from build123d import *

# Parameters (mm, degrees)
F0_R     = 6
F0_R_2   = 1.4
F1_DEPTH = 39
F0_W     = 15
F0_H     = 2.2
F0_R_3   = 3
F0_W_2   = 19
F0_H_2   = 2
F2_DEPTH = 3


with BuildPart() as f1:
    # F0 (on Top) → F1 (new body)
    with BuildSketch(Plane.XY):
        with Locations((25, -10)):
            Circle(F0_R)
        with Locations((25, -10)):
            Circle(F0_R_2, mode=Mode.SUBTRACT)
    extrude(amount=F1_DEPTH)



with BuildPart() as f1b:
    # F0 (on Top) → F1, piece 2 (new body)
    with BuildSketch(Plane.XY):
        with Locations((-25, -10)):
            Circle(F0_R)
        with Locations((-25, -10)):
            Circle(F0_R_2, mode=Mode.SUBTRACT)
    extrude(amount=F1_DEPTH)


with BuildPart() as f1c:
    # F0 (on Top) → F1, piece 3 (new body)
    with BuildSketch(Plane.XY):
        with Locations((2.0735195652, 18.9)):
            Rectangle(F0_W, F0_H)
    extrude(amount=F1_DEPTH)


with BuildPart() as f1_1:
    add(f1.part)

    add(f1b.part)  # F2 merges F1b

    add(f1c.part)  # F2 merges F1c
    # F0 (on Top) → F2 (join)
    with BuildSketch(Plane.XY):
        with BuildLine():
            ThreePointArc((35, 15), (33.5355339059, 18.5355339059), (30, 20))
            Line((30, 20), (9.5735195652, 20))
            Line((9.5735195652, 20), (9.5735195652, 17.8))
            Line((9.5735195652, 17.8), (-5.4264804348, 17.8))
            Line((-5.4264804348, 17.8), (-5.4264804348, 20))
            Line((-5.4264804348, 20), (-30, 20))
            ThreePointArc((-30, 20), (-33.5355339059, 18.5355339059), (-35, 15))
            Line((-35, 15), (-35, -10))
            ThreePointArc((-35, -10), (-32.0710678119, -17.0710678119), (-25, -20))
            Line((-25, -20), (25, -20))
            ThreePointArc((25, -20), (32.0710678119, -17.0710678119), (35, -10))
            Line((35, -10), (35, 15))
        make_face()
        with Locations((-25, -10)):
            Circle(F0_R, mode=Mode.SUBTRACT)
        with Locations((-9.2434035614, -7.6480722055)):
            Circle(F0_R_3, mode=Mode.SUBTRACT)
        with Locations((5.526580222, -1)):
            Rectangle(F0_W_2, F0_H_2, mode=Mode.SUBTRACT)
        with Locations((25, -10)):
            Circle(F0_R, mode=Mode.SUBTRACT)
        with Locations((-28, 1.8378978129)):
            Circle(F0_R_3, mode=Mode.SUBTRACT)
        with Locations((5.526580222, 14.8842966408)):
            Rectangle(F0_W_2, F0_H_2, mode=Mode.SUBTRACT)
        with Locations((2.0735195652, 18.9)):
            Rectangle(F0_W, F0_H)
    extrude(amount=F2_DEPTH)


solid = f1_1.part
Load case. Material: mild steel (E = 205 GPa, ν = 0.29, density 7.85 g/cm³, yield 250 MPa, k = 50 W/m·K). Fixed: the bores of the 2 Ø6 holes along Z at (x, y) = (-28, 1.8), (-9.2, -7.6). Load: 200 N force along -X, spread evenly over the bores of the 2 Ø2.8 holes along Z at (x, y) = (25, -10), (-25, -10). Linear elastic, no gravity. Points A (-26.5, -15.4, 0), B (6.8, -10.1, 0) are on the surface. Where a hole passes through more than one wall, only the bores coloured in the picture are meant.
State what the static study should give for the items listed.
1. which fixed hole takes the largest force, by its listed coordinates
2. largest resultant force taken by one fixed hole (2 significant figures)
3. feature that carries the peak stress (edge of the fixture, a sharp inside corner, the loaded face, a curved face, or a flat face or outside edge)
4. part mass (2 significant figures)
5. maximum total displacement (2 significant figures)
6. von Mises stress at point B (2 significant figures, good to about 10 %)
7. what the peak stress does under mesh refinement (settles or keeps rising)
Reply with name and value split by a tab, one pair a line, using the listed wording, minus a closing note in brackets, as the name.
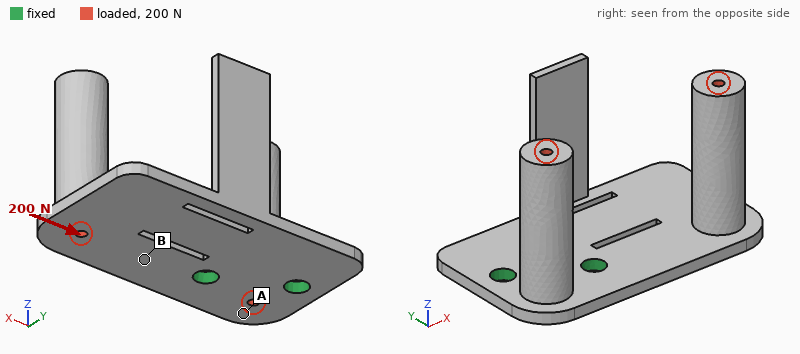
which fixed hole takes the largest force, by its listed coordinates	(-9.2, -7.6)
largest resultant force taken by one fixed hole	200 N
feature that carries the peak stress	edge of the fixture
part mass	130 g
maximum total displacement	0.16 mm
von Mises stress at point B	32 MPa
what the peak stress does under mesh refinement	keeps rising
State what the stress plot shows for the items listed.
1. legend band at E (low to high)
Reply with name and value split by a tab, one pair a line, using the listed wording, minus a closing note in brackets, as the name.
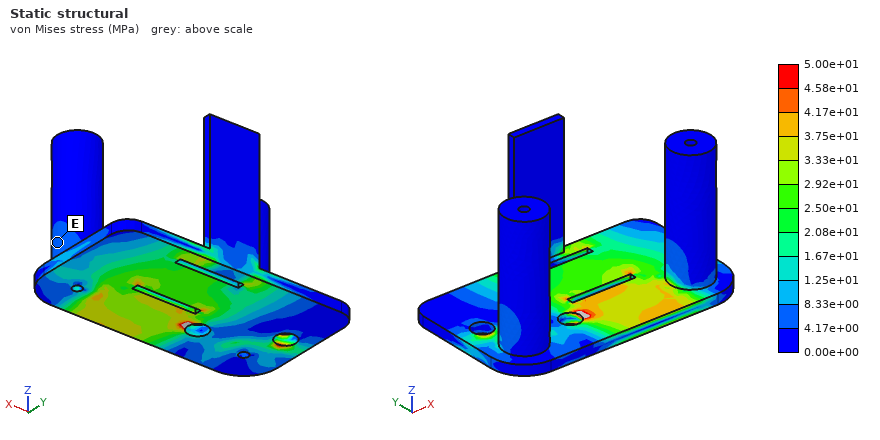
legend band at E	4.17e+00 to 8.33e+00 MPa
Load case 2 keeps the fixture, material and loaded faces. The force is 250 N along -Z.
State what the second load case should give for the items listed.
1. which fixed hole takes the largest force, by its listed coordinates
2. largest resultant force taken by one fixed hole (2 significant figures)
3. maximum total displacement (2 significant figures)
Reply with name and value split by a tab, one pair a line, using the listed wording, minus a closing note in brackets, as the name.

which fixed hole takes the largest force, by its listed coordinates	(-9.2, -7.6)
largest resultant force taken by one fixed hole	240 N
maximum total displacement	0.21 mm
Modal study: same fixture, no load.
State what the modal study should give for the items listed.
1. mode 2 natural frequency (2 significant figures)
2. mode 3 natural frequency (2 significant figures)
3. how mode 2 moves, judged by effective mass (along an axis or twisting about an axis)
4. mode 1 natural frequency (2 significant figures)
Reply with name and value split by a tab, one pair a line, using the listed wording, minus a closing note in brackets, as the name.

mode 2 natural frequency	880 Hz
mode 3 natural frequency	1100 Hz
how mode 2 moves, judged by effective mass	along Y
mode 1 natural frequency	610 Hz
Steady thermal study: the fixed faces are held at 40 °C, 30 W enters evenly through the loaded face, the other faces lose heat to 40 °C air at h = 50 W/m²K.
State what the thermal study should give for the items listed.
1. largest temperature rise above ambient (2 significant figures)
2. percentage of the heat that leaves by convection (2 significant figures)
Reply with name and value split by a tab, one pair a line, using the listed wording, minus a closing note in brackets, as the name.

largest temperature rise above ambient	79 K
percentage of the heat that leaves by convection	48 %
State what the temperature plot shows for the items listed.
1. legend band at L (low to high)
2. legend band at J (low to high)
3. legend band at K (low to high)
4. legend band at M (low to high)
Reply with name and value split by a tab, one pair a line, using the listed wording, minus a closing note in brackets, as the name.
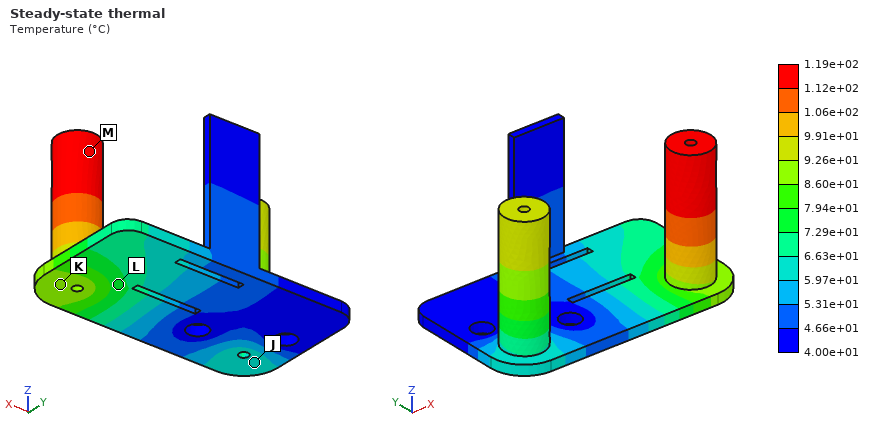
legend band at L	7.29e+01 to 7.94e+01 °C
legend band at J	5.97e+01 to 6.63e+01 °C
legend band at K	8.60e+01 to 9.26e+01 °C
legend band at M	1.12e+02 to 1.19e+02 °C
